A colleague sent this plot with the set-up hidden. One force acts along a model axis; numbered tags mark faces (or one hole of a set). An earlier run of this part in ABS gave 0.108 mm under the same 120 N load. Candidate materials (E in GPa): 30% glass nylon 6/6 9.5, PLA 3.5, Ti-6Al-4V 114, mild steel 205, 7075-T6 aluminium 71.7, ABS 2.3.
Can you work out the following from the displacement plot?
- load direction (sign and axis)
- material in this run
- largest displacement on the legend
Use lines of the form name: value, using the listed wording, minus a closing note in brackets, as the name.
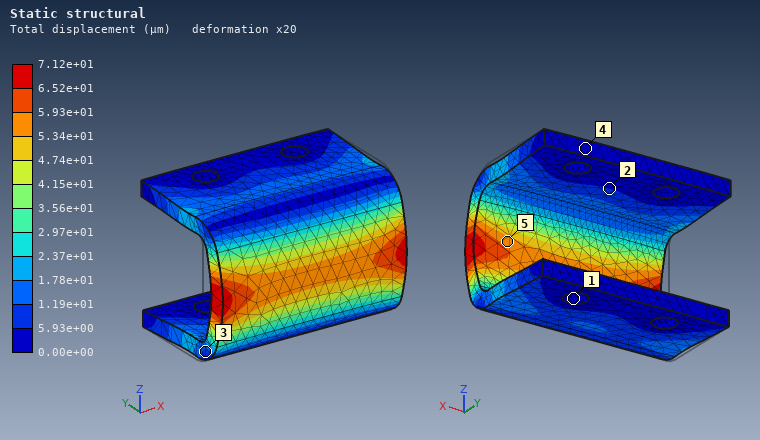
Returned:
load direction: -Y
material in this run: PLA
largest displacement on the legend: 7.12e+01 µm
